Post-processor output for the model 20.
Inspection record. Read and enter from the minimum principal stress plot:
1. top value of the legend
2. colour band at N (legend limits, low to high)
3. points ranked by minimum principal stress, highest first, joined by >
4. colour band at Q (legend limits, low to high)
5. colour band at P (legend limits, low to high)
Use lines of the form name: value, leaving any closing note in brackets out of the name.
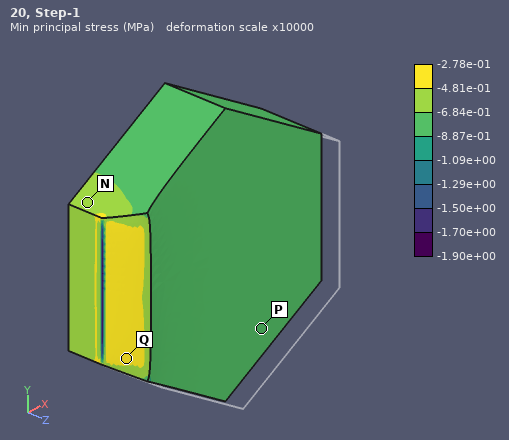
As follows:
top value of the legend: -2.78e-01 MPa
colour band at N: -6.84e-01 to -4.81e-01 MPa
points ranked by minimum principal stress, highest first, joined by >: Q > N > P
colour band at Q: -4.81e-01 to -2.78e-01 MPa
colour band at P: -8.87e-01 to -6.84e-01 MPa
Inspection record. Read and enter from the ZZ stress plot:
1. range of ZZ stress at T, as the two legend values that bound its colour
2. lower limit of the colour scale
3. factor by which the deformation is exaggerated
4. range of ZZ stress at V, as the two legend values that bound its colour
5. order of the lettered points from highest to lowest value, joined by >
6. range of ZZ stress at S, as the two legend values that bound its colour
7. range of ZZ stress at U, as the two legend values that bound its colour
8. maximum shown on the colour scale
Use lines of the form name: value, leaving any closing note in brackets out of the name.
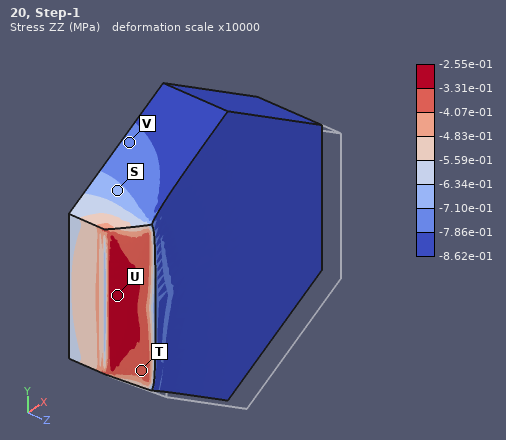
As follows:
range of ZZ stress at T, as the two legend values that bound its colour: -4.07e-01 to -3.31e-01 MPa
lower limit of the colour scale: -8.62e-01 MPa
factor by which the deformation is exaggerated: 10000
range of ZZ stress at V, as the two legend values that bound its colour: -7.86e-01 to -7.10e-01 MPa
order of the lettered points from highest to lowest value, joined by >: U > T > S > V
range of ZZ stress at S, as the two legend values that bound its colour: -7.10e-01 to -6.34e-01 MPa
range of ZZ stress at U, as the two legend values that bound its colour: -3.31e-01 to -2.55e-01 MPa
maximum shown on the colour scale: -2.55e-01 MPa
